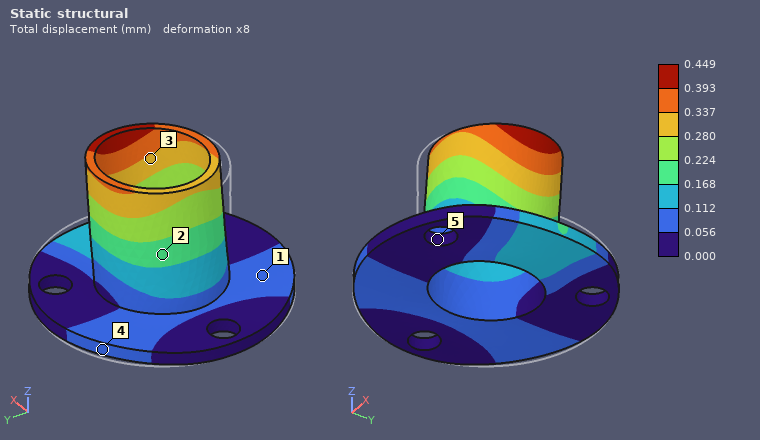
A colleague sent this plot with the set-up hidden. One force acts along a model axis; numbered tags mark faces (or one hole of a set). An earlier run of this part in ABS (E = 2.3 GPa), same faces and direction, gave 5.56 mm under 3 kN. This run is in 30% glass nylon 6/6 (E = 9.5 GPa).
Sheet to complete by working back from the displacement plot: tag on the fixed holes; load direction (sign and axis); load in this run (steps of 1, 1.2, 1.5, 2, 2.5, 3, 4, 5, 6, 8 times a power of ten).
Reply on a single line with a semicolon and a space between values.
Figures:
5; +X; 1 kN
